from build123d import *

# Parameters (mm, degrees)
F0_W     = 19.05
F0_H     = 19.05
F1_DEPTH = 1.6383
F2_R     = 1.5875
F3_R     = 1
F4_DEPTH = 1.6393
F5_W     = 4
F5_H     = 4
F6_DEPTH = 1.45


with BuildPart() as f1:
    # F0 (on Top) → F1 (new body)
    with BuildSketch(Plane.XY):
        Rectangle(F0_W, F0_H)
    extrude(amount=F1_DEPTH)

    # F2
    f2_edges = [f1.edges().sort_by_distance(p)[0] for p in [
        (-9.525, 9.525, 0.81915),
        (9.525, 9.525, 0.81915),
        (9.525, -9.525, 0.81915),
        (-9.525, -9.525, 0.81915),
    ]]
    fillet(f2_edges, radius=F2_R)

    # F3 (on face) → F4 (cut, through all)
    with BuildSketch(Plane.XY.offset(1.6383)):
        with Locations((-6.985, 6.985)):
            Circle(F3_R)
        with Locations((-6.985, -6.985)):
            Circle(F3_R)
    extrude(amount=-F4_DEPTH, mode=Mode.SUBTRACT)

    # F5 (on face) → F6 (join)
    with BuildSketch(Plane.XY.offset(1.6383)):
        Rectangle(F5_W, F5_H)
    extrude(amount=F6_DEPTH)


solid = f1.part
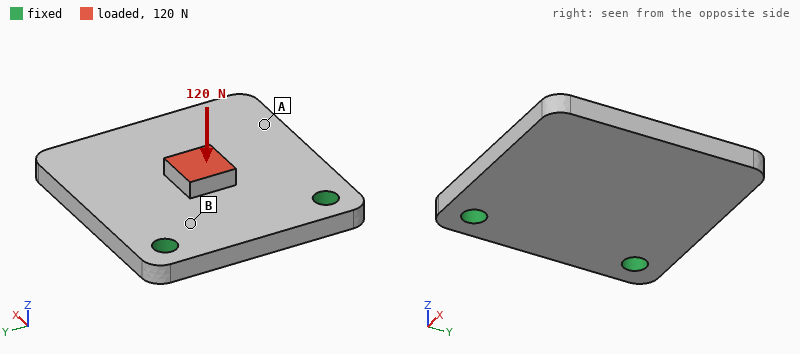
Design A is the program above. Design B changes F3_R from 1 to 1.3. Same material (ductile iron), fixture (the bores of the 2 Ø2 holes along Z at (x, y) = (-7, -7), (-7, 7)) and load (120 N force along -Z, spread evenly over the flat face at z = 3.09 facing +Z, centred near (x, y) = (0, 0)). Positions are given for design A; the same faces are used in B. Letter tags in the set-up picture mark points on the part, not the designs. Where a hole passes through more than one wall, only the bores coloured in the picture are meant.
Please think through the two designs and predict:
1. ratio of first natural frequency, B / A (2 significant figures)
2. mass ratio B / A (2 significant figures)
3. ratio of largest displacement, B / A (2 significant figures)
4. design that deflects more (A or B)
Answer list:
1.1
0.99
0.87
A
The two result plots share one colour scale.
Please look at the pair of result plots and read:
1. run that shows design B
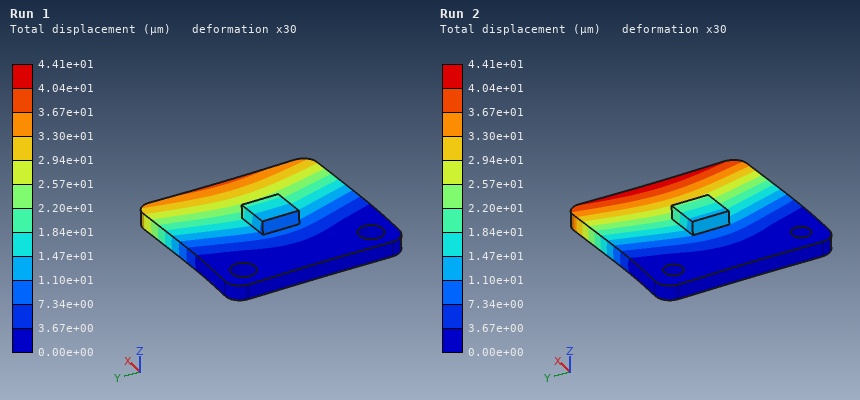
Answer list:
Run 1
